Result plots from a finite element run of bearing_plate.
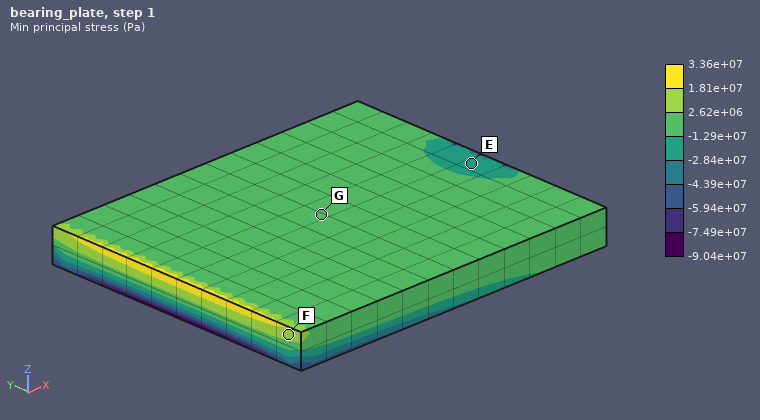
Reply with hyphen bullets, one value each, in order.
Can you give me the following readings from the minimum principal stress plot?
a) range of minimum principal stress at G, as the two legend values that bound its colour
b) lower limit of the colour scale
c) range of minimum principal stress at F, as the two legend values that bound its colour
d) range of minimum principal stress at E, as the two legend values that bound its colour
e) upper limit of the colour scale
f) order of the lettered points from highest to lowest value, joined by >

- -1.29e+07 to 2.62e+06 Pa
- -9.04e+07 Pa
- 2.62e+06 to 1.81e+07 Pa
- -2.84e+07 to -1.29e+07 Pa
- 3.36e+07 Pa
- F > G > E
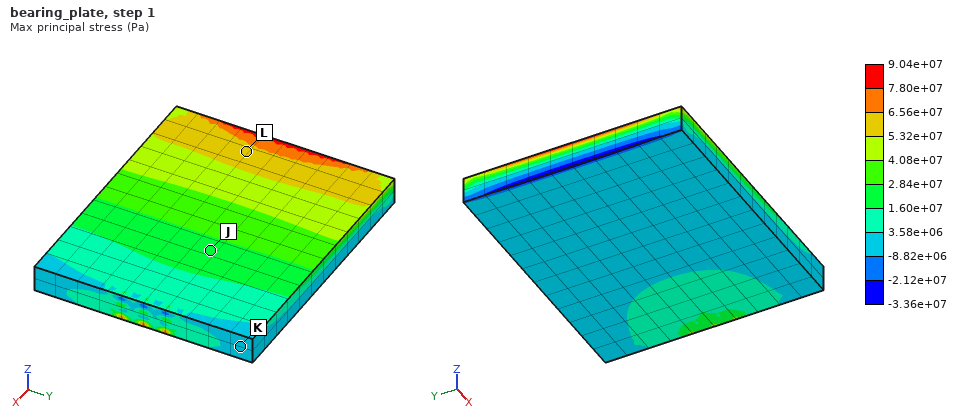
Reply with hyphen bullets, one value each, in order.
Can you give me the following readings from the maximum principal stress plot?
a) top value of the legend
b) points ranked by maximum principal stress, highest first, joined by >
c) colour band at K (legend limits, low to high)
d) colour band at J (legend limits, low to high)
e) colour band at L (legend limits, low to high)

- 9.04e+07 Pa
- L > J > K
- -8.82e+06 to 3.58e+06 Pa
- 1.60e+07 to 2.84e+07 Pa
- 5.32e+07 to 6.56e+07 Pa
